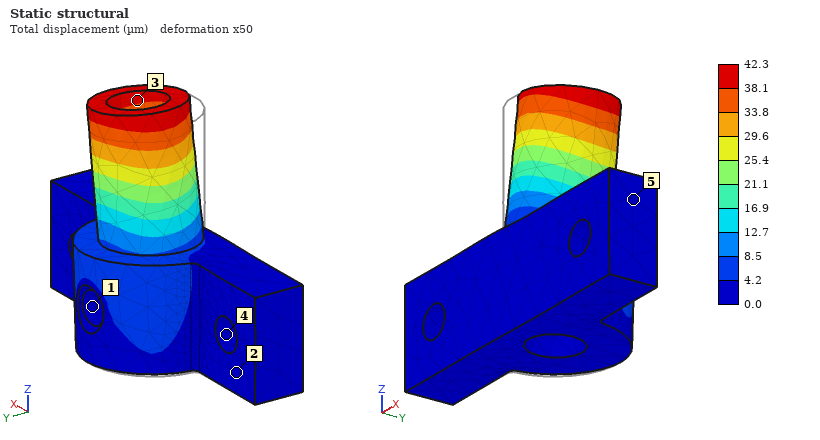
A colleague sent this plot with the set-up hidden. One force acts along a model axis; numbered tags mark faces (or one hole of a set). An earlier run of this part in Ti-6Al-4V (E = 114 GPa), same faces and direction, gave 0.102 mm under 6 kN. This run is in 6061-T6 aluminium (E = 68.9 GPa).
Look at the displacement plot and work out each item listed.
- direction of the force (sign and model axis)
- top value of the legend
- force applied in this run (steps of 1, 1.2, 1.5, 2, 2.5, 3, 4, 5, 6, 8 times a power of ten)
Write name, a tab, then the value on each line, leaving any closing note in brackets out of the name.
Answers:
direction of the force	+X
top value of the legend	42.3 µm
force applied in this run	1.5 kN
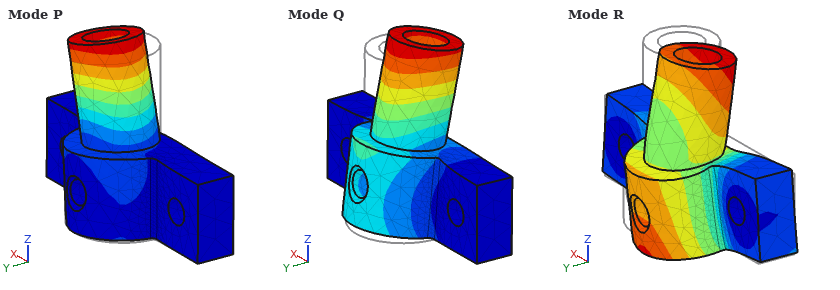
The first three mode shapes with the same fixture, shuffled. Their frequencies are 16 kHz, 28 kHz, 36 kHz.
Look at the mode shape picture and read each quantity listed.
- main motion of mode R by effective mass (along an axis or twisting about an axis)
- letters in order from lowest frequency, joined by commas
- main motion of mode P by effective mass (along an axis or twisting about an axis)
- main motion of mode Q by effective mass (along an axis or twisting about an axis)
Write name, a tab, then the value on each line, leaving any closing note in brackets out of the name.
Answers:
main motion of mode R by effective mass	along Z
letters in order from lowest frequency, joined by commas	Q, P, R
main motion of mode P by effective mass	along X
main motion of mode Q by effective mass	along Y
